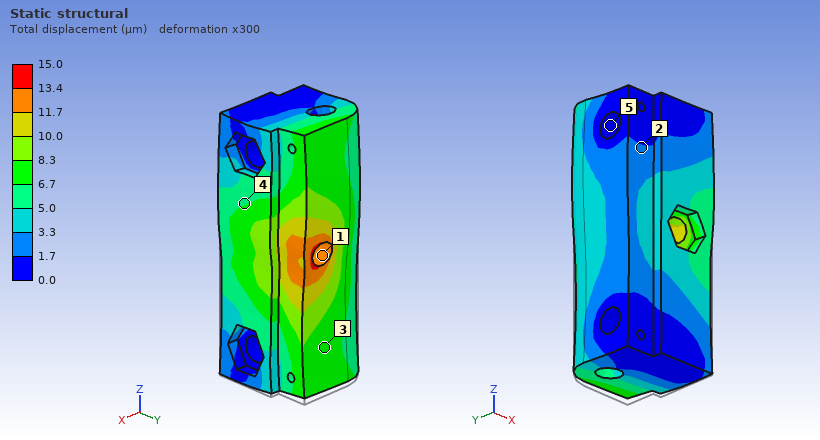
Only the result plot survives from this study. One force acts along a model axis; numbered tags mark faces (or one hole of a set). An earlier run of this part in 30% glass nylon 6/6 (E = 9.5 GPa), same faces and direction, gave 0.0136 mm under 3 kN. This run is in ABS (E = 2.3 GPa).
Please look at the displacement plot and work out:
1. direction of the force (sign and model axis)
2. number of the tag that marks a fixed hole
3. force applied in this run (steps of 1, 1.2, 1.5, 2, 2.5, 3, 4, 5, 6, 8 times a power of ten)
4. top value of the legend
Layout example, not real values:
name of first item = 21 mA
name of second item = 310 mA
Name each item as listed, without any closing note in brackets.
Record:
direction of the force = +Z
number of the tag that marks a fixed hole = 5
force applied in this run = 800 N
top value of the legend = 15.0 µm
